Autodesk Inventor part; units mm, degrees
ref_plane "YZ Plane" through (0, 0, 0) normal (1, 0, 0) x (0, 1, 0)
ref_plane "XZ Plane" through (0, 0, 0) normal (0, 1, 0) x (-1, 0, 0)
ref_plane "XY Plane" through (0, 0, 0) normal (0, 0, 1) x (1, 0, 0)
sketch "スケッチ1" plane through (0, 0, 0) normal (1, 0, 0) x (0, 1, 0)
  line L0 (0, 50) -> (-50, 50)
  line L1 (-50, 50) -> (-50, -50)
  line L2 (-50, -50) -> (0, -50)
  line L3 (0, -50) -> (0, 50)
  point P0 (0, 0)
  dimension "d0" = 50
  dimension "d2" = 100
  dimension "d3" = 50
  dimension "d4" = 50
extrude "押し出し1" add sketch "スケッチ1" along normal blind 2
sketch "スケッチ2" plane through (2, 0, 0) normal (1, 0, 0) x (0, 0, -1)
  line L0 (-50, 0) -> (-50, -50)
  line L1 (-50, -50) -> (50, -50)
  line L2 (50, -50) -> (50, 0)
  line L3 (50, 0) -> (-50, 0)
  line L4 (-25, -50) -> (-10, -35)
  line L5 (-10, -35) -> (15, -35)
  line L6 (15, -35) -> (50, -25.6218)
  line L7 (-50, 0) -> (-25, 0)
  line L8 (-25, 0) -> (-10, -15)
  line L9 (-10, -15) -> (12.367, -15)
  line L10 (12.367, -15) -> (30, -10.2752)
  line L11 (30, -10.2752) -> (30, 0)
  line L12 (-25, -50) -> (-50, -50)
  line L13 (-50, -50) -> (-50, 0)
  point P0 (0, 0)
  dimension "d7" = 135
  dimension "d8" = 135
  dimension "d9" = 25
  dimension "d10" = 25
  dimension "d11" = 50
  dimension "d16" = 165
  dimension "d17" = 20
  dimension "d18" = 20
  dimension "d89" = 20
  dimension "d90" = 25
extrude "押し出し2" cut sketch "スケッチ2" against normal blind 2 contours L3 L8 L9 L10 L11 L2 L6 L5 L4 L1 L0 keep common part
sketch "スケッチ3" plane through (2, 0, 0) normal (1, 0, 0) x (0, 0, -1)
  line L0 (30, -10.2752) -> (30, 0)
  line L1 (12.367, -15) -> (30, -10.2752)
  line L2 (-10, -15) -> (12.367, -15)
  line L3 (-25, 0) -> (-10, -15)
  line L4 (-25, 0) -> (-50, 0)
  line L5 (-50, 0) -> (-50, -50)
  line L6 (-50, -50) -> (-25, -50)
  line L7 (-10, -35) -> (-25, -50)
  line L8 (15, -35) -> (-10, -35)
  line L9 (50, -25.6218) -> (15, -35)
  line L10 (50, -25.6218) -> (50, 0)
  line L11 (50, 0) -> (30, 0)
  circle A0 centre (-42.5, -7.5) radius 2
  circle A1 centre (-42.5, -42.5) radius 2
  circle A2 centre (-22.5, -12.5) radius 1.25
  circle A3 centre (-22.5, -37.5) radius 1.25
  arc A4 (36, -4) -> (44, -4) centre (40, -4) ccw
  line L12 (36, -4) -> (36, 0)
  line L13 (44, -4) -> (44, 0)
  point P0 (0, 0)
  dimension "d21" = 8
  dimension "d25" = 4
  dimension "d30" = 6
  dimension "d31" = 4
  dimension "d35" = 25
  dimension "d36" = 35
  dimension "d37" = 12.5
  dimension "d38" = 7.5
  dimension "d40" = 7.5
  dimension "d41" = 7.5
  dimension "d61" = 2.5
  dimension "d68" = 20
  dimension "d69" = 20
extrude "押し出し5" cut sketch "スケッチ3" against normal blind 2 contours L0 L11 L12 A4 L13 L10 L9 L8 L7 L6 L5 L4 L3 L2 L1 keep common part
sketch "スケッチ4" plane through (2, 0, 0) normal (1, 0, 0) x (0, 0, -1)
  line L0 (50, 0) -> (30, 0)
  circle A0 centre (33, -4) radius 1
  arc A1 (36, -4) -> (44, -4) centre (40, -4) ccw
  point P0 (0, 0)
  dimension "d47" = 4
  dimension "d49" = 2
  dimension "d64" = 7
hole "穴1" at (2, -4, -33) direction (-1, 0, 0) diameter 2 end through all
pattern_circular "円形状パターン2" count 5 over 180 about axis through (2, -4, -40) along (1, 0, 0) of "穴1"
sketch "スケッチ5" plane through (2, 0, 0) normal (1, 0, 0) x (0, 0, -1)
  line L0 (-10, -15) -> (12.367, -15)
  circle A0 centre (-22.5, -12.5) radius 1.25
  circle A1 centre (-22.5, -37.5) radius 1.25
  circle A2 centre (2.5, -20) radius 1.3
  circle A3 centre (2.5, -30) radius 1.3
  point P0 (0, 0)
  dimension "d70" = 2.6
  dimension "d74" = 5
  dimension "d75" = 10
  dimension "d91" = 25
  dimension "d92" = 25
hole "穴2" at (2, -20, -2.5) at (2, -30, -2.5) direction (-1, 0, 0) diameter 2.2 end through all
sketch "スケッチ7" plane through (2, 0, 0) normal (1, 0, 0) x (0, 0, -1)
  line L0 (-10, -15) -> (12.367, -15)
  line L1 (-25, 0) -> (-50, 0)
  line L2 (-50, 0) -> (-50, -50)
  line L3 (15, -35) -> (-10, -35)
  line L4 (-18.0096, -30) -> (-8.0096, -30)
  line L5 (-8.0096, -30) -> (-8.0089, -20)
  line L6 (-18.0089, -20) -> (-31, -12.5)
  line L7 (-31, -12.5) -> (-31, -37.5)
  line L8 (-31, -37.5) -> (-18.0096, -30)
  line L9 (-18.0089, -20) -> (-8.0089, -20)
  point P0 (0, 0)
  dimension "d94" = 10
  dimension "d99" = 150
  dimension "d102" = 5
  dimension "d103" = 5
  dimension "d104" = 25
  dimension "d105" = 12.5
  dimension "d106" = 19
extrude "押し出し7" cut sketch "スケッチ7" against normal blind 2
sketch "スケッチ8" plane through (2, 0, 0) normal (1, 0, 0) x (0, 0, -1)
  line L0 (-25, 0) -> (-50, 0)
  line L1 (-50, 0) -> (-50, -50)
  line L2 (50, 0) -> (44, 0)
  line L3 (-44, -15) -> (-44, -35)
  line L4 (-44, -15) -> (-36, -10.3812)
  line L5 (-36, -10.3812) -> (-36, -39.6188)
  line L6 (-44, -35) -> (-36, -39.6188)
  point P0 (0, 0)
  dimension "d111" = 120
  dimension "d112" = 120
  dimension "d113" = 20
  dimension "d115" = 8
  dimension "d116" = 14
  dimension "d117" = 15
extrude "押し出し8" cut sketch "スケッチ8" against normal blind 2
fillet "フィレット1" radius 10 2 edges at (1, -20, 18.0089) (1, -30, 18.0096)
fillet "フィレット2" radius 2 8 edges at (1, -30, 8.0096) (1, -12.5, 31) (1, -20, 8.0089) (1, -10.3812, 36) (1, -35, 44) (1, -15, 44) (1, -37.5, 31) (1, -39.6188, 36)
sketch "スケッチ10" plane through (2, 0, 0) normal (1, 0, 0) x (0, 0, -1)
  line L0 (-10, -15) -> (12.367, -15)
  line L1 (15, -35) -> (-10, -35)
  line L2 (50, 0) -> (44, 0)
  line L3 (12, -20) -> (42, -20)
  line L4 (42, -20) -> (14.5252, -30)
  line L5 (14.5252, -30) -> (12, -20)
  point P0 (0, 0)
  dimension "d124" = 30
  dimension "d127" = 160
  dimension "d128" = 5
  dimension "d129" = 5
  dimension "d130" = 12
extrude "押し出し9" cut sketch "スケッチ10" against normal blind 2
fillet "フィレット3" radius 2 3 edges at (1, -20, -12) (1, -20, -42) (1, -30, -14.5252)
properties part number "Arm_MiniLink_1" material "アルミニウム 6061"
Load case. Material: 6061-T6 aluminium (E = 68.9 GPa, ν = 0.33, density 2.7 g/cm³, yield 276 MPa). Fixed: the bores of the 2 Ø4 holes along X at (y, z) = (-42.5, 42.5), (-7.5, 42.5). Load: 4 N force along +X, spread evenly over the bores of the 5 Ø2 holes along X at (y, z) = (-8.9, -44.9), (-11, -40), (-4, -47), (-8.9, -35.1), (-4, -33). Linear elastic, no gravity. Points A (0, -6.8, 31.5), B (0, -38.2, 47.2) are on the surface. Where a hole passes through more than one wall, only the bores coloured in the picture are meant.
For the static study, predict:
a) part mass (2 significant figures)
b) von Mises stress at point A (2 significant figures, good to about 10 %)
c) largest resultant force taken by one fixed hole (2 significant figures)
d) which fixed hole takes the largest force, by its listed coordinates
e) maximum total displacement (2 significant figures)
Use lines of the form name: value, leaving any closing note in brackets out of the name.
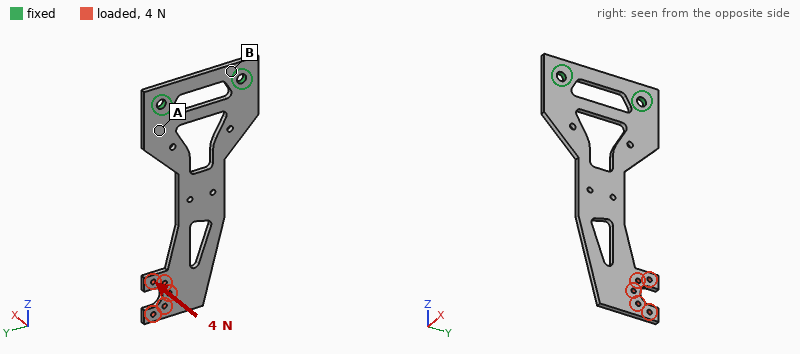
part mass: 13 g
von Mises stress at point A: 16 MPa
largest resultant force taken by one fixed hole: 3.6 N
which fixed hole takes the largest force, by its listed coordinates: (-7.5, 42.5)
maximum total displacement: 1.1 mm
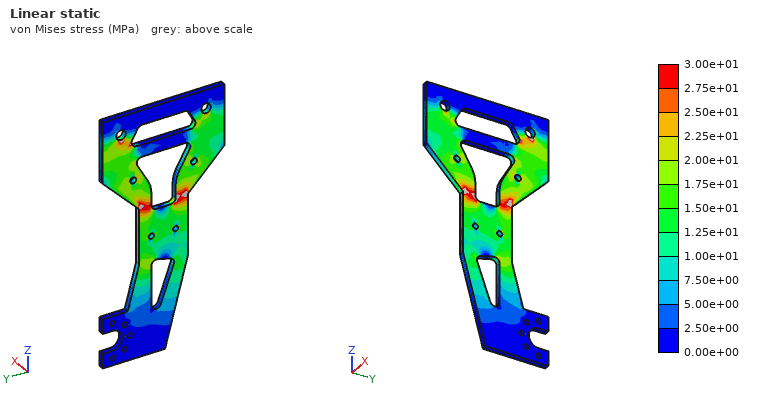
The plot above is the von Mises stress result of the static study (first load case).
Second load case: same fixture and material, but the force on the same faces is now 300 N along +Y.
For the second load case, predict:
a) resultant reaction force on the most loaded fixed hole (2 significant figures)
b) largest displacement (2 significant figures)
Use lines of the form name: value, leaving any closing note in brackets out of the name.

resultant reaction force on the most loaded fixed hole: 730 N
largest displacement: 0.56 mm
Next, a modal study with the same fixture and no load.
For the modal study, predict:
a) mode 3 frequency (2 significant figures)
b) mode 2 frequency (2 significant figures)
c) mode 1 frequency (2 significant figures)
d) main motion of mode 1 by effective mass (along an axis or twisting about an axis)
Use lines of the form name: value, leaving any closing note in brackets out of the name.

mode 3 frequency: 1400 Hz
mode 2 frequency: 1000 Hz
mode 1 frequency: 190 Hz
main motion of mode 1 by effective mass: along X
